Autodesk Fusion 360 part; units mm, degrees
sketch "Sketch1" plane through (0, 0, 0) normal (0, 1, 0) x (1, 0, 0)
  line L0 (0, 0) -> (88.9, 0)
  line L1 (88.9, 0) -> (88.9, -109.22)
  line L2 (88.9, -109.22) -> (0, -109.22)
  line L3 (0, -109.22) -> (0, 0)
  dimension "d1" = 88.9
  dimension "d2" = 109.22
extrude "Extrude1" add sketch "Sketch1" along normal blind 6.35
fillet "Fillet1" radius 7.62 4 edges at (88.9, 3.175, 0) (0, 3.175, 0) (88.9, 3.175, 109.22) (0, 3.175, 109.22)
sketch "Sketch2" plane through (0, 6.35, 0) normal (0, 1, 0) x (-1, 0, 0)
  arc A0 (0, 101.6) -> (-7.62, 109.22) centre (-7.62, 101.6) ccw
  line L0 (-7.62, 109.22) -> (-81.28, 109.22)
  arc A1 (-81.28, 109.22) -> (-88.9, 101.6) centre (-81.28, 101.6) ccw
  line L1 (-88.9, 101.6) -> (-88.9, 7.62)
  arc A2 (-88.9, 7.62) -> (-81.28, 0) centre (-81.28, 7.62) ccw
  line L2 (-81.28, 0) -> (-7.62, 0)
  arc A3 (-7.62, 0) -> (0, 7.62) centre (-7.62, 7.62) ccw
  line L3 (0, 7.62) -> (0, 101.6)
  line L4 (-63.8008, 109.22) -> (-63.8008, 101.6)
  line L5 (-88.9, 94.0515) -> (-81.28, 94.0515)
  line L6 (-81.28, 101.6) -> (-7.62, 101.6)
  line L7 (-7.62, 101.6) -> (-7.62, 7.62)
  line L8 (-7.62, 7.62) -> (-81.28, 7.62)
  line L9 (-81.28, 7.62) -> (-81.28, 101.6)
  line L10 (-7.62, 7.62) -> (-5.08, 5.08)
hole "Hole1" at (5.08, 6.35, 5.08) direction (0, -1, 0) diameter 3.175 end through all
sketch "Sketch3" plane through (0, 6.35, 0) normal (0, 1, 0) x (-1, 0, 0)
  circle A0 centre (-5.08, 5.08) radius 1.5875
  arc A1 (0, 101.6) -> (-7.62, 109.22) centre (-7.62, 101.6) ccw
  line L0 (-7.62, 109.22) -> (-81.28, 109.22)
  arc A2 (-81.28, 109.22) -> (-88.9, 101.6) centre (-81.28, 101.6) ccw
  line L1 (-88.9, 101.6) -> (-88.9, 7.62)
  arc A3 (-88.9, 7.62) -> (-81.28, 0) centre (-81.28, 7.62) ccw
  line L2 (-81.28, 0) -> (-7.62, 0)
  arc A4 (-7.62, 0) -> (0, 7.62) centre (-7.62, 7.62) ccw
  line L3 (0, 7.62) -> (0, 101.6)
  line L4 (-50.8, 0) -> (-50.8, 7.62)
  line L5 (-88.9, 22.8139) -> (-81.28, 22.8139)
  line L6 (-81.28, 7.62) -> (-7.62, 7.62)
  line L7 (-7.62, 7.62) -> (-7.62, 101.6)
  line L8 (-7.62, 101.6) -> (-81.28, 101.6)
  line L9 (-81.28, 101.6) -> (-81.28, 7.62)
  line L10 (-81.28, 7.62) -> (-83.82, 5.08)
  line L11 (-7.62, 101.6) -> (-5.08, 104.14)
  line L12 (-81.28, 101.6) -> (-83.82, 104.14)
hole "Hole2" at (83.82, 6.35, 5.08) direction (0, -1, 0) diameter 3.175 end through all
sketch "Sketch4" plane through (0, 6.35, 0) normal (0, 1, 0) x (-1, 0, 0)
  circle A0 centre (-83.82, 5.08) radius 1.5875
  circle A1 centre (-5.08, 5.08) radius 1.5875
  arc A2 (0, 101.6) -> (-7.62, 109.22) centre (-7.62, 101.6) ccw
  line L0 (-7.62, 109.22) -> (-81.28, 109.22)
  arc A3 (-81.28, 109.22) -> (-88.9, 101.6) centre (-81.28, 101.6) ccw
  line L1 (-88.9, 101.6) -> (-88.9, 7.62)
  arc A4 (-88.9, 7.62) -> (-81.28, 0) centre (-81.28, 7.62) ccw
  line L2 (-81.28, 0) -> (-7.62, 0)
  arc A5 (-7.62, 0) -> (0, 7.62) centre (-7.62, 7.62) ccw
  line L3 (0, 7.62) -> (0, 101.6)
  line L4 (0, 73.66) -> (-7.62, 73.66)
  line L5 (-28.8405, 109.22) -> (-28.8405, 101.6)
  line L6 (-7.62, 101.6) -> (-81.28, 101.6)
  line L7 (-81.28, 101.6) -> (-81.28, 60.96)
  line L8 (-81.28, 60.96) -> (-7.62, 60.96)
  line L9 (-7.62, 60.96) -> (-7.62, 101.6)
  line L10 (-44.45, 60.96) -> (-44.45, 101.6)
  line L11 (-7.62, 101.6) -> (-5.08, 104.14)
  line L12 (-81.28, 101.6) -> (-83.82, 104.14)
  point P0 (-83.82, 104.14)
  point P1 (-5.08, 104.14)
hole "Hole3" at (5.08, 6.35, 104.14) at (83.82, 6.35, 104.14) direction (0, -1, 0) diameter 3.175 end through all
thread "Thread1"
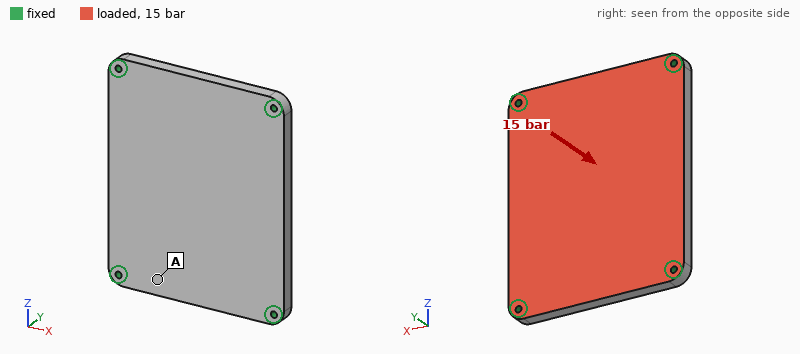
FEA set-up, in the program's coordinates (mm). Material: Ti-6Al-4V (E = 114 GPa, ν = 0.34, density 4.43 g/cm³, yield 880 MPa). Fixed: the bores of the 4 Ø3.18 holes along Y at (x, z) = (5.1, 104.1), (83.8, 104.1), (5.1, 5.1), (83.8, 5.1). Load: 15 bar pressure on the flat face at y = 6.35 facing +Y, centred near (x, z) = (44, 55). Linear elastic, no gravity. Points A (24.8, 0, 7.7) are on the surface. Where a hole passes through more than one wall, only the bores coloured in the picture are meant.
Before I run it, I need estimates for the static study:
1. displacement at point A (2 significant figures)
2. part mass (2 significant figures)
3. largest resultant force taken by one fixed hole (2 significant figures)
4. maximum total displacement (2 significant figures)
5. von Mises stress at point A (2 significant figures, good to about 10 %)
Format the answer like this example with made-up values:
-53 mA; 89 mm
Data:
0.099 mm; 270 g; 3.6 kN; 0.37 mm; 44 MPa
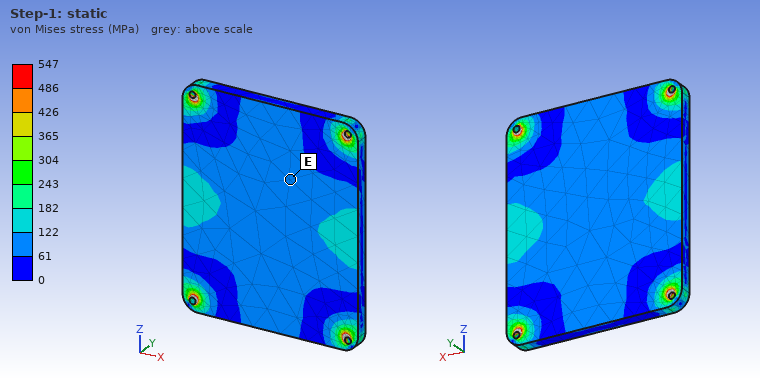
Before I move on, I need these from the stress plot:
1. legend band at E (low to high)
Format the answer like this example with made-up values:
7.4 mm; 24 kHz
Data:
61 to 122 MPa
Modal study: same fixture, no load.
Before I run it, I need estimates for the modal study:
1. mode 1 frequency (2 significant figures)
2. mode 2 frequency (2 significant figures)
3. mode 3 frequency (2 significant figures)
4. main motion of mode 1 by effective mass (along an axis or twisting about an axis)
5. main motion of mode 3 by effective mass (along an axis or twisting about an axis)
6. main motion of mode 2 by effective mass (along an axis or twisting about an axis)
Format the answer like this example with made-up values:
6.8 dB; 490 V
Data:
2300 Hz; 3700 Hz; 4700 Hz; along Y; twisting about X; twisting about Z
